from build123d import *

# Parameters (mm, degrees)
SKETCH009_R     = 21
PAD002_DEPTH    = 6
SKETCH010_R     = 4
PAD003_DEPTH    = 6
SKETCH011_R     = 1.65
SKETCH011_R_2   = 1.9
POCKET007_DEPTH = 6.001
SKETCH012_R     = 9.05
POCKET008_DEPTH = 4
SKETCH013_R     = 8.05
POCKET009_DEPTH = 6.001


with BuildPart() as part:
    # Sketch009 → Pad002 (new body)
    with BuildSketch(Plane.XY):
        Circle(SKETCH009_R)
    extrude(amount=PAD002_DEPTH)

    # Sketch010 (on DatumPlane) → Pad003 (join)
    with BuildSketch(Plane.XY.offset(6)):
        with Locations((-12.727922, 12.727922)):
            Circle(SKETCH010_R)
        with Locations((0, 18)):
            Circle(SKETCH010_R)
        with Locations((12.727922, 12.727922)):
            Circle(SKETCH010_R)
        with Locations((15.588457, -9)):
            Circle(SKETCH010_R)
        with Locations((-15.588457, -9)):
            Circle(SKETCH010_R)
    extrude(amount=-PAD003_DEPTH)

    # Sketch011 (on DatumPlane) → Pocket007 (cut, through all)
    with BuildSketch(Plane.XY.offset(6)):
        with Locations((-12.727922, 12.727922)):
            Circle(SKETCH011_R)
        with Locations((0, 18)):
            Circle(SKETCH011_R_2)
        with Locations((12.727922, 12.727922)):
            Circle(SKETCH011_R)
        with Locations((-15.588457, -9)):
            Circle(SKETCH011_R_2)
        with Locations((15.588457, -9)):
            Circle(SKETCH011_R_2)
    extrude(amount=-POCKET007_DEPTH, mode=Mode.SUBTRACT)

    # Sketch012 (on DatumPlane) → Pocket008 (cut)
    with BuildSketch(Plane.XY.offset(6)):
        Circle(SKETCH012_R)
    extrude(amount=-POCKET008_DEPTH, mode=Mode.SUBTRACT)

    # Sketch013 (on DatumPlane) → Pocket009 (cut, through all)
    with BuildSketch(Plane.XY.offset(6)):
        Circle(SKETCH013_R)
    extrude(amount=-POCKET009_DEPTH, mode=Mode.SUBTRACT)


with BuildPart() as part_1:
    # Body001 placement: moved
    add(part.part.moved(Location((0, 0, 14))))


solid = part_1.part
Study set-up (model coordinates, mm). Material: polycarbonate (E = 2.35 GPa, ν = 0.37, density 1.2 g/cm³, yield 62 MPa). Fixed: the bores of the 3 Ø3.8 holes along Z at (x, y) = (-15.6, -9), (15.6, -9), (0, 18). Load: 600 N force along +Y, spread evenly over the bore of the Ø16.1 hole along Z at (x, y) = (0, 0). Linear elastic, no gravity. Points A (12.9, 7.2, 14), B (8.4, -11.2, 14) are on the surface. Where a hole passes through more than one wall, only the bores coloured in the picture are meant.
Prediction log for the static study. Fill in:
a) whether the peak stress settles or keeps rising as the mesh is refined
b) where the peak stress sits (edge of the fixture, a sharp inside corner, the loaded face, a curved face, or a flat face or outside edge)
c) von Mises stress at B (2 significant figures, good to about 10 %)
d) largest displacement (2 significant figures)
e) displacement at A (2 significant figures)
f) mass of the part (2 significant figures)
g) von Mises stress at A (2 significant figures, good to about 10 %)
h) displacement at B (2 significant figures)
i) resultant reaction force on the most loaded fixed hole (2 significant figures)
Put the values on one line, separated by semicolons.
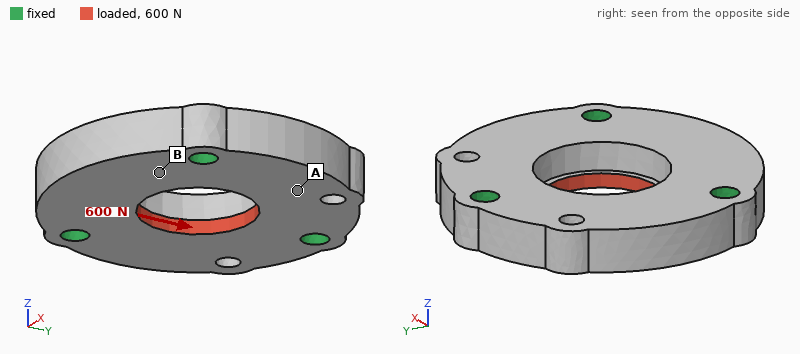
keeps rising; edge of the fixture; 4.3 MPa; 53 µm; 21 µm; 8.0 g; 1.5 MPa; 25 µm; 210 N
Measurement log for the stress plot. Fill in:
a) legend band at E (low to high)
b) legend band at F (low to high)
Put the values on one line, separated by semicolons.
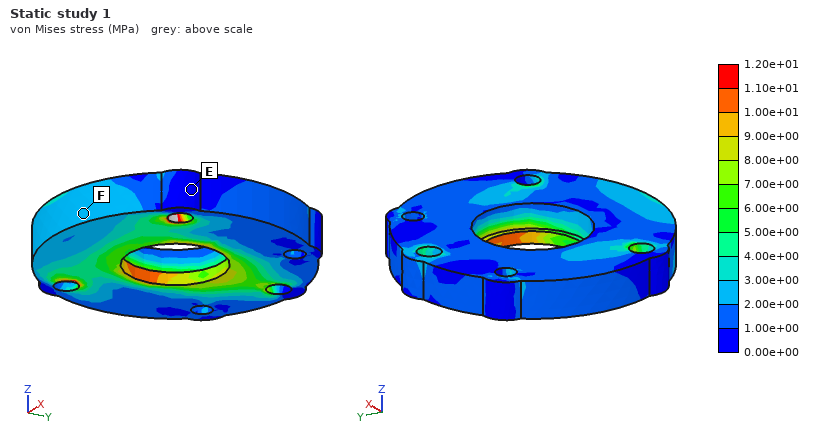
0.00e+00 to 1.00e+00 MPa; 2.00e+00 to 3.00e+00 MPa
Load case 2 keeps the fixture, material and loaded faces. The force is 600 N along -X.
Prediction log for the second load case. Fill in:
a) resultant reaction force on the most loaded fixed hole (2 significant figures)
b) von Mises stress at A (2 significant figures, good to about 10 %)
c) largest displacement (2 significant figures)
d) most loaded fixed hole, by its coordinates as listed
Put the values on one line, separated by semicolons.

220 N; 2.6 MPa; 49 µm; (0, 18)
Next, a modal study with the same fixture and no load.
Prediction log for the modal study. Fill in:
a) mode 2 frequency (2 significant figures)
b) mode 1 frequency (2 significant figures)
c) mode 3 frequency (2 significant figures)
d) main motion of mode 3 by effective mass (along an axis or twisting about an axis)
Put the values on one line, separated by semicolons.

5500 Hz; 5500 Hz; 6200 Hz; along Z
